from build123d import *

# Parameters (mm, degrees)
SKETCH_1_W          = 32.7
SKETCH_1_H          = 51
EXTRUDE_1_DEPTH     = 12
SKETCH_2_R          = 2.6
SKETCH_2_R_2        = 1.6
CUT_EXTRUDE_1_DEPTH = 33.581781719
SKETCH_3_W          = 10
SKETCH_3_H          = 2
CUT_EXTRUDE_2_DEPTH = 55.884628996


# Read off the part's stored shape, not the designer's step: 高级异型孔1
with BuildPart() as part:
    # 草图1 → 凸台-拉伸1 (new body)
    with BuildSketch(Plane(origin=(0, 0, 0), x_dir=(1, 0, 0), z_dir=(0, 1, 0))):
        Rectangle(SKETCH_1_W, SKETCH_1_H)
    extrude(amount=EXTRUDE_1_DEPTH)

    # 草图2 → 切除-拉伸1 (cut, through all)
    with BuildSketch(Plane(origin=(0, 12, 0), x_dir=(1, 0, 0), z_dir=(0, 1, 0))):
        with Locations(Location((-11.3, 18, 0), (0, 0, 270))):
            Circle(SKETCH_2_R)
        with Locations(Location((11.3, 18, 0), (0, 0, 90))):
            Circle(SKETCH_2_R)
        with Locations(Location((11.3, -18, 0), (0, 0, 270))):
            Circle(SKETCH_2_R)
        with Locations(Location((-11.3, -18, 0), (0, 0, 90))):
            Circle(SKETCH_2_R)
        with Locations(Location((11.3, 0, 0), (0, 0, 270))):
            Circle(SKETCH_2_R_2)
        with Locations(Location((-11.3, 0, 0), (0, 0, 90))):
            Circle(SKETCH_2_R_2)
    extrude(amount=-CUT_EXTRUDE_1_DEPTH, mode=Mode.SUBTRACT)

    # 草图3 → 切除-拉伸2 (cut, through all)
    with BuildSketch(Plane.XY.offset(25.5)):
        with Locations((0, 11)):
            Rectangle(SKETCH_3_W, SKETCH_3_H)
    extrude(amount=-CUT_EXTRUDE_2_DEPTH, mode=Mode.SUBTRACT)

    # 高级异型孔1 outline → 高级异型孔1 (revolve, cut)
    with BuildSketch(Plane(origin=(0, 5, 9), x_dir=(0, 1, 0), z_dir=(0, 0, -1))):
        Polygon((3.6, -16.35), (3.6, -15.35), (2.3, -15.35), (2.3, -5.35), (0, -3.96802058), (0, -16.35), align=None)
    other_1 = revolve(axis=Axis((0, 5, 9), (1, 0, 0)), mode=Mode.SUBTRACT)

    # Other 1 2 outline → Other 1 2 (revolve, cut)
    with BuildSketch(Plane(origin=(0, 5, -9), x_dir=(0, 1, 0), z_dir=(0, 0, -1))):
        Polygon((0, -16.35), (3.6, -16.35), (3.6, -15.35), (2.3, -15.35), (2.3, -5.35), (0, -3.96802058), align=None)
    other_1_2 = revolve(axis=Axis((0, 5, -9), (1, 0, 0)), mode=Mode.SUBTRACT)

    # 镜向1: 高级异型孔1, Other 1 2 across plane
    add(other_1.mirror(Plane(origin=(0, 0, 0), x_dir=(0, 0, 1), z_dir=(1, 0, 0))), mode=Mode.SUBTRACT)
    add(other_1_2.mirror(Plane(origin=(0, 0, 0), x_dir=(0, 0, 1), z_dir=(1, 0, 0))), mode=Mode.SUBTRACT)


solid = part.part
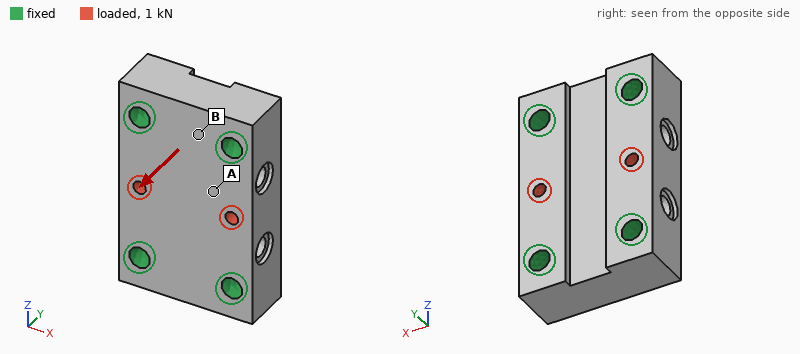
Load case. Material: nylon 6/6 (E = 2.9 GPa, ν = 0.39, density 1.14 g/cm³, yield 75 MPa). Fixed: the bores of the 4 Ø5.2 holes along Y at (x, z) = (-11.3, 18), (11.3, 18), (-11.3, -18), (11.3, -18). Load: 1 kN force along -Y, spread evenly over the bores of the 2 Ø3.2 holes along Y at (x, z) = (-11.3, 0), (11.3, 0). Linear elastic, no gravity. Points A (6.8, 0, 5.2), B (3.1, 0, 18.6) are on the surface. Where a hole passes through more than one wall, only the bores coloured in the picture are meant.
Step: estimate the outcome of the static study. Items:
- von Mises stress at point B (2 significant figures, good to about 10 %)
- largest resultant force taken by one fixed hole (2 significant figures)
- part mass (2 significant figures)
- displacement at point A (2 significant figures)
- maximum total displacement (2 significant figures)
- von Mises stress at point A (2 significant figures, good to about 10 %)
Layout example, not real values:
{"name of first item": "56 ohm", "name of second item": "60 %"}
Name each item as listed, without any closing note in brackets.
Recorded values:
{"von Mises stress at point B": "1.7 MPa", "largest resultant force taken by one fixed hole": "250 N", "part mass": "19 g", "displacement at point A": "43 µm", "maximum total displacement": "72 µm", "von Mises stress at point A": "4.3 MPa"}
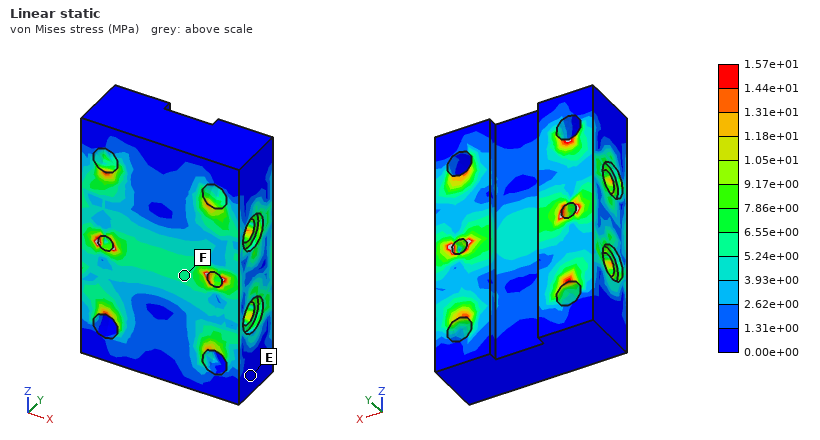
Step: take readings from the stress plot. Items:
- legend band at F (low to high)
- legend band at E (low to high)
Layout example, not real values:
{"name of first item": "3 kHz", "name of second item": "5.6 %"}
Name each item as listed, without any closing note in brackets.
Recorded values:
{"legend band at F": "5.24e+00 to 6.55e+00 MPa", "legend band at E": "0.00e+00 to 1.31e+00 MPa"}
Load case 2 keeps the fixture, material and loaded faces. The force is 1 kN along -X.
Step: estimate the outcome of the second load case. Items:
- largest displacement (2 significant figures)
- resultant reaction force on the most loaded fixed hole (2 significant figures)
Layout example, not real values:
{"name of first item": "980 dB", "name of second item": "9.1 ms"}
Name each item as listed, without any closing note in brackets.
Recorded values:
{"largest displacement": "38 µm", "resultant reaction force on the most loaded fixed hole": "290 N"}
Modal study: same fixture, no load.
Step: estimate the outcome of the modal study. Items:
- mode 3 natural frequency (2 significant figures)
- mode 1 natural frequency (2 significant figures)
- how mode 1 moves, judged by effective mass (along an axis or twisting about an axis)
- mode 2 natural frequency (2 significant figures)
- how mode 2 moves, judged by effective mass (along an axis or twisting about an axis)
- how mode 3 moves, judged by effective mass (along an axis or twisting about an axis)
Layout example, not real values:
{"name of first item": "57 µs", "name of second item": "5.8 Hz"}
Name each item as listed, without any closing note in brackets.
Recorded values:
{"mode 3 natural frequency": "12 kHz", "mode 1 natural frequency": "8900 Hz", "how mode 1 moves, judged by effective mass": "along Y", "mode 2 natural frequency": "10 kHz", "how mode 2 moves, judged by effective mass": "twisting about Z", "how mode 3 moves, judged by effective mass": "along X"}
